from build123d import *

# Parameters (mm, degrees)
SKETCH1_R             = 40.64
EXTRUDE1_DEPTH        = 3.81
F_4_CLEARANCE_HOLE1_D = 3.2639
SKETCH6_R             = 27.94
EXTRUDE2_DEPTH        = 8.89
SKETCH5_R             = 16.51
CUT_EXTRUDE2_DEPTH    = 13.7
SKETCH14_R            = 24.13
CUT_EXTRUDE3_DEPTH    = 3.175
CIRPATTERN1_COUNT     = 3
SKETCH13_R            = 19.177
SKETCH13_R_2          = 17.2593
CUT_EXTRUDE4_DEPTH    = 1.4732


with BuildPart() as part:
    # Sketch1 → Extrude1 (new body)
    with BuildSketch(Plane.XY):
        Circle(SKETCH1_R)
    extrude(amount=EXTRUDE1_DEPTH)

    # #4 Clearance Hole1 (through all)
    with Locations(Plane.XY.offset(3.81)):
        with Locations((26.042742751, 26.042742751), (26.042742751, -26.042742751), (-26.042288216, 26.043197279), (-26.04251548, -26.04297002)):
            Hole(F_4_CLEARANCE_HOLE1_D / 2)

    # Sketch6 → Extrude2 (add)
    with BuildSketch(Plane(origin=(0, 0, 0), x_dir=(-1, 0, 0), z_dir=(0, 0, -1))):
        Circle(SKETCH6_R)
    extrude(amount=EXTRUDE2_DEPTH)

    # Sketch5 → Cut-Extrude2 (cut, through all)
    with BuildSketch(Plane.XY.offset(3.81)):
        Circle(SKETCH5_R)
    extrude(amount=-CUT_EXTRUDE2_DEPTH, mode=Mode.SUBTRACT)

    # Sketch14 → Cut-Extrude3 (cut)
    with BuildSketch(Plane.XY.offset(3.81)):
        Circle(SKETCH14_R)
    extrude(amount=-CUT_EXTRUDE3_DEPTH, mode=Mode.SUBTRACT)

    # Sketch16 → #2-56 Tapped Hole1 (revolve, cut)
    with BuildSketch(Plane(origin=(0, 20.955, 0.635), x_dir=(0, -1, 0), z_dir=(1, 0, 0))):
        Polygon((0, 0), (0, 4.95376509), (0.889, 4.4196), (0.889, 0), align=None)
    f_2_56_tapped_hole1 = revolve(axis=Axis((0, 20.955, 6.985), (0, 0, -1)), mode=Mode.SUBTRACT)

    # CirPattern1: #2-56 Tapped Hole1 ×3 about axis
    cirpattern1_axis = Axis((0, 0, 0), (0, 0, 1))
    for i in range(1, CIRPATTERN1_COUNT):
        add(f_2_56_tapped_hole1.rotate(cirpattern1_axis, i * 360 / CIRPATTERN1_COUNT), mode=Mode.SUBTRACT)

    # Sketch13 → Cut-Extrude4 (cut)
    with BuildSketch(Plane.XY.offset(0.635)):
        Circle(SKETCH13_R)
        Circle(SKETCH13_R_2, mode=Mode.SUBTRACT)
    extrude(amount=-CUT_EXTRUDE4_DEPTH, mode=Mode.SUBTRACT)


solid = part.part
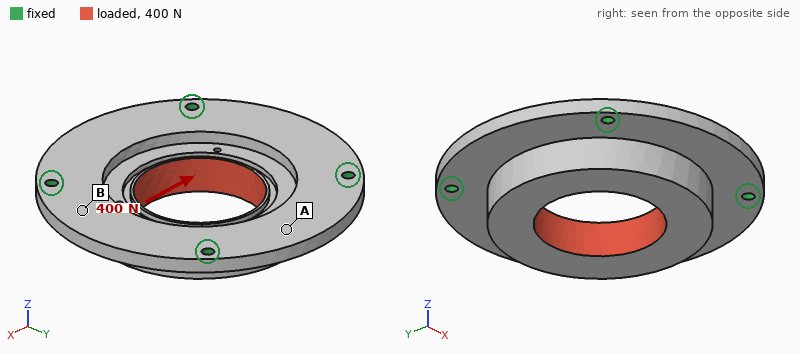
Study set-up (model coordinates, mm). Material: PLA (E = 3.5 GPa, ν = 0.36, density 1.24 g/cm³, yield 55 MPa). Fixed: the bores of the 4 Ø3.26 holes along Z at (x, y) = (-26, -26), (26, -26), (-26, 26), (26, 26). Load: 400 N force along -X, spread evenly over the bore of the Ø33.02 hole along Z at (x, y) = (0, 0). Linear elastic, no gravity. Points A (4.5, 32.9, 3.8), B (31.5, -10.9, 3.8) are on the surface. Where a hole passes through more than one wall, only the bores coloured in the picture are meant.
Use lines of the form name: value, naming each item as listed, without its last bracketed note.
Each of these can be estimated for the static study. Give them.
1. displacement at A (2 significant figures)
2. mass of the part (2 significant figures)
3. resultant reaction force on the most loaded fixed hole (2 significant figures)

displacement at A: 5.6 µm
mass of the part: 34 g
resultant reaction force on the most loaded fixed hole: 100 N
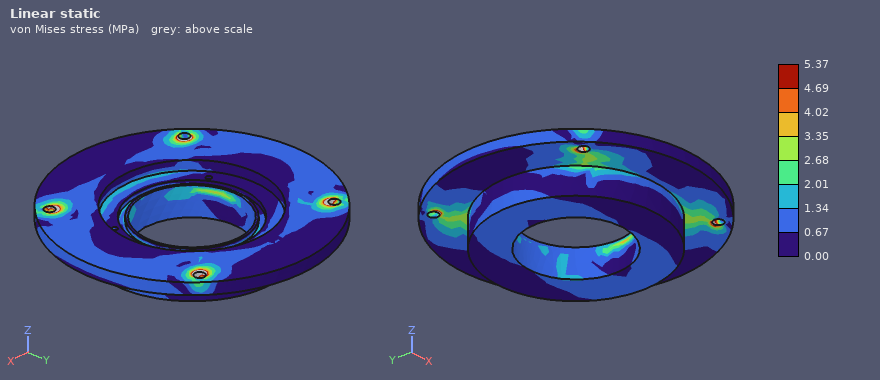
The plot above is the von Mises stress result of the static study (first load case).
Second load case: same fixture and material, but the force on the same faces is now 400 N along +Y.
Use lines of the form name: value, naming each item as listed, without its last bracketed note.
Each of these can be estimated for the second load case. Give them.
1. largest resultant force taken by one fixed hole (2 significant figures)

largest resultant force taken by one fixed hole: 100 N
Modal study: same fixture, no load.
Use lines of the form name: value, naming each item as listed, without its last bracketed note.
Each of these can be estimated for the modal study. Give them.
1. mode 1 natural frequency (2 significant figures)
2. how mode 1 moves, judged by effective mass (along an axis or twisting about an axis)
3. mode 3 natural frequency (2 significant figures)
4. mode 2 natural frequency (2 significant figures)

mode 1 natural frequency: 2300 Hz
how mode 1 moves, judged by effective mass: along Z
mode 3 natural frequency: 2600 Hz
mode 2 natural frequency: 2600 Hz
